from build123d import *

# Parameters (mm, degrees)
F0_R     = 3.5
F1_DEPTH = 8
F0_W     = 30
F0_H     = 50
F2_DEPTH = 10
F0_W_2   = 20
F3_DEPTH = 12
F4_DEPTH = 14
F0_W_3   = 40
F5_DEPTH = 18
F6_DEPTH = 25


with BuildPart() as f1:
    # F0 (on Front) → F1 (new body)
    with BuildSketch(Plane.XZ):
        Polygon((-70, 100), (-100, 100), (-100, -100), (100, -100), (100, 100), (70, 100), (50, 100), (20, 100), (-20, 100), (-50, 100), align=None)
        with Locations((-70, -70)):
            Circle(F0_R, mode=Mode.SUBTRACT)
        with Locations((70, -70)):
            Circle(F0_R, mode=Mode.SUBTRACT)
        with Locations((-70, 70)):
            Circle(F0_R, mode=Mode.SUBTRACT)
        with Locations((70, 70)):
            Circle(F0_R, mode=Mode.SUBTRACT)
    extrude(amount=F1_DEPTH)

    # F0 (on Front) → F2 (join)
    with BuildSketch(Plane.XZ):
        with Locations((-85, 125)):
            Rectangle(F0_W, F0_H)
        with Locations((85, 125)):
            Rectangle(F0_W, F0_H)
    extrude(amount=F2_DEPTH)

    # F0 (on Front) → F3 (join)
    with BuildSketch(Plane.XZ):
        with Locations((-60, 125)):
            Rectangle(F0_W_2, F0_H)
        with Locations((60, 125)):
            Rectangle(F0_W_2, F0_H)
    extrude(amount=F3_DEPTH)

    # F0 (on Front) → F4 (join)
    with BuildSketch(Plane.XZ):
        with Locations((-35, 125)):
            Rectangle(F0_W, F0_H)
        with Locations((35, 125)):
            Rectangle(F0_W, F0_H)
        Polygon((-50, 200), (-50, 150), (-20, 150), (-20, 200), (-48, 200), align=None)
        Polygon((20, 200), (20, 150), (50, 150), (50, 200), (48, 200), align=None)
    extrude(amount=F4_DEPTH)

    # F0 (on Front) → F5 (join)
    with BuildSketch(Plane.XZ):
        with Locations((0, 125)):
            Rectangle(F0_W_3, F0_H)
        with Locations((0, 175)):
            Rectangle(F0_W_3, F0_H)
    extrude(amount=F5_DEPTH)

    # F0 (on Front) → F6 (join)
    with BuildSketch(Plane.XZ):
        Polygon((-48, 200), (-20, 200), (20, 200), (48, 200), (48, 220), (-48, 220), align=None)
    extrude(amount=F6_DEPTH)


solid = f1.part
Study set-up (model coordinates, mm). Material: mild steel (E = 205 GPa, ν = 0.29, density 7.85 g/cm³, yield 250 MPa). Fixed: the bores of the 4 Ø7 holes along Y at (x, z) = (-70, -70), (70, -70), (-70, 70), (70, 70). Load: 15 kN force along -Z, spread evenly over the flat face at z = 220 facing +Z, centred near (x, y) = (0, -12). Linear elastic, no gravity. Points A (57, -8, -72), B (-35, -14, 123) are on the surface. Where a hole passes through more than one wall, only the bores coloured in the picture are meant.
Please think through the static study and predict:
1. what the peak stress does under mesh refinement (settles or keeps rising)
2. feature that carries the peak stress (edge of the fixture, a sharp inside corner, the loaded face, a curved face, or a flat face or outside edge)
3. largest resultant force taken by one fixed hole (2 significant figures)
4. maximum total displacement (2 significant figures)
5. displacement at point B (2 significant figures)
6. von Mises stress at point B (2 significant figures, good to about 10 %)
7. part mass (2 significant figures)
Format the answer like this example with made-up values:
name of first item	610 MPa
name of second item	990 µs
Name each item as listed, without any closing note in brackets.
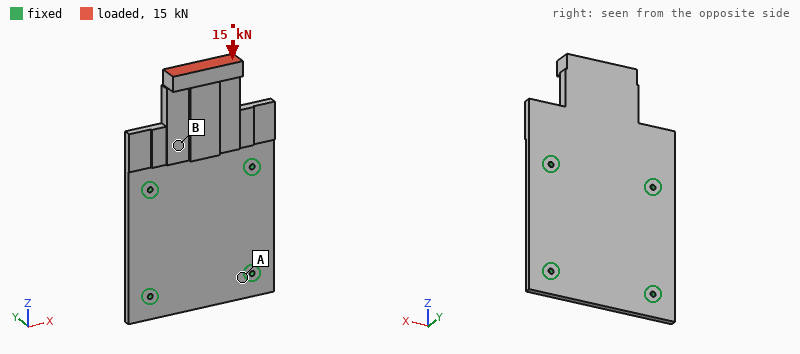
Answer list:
what the peak stress does under mesh refinement	keeps rising
feature that carries the peak stress	edge of the fixture
largest resultant force taken by one fixed hole	5.8 kN
maximum total displacement	0.50 mm
displacement at point B	0.13 mm
von Mises stress at point B	25 MPa
part mass	4.5 kg
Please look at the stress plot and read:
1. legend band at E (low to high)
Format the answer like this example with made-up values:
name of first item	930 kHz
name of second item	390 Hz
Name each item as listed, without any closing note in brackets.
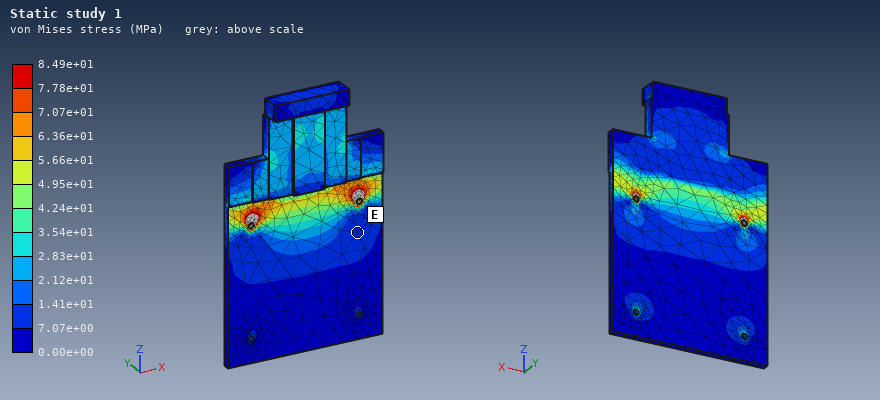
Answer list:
legend band at E	7.07e+00 to 1.41e+01 MPa
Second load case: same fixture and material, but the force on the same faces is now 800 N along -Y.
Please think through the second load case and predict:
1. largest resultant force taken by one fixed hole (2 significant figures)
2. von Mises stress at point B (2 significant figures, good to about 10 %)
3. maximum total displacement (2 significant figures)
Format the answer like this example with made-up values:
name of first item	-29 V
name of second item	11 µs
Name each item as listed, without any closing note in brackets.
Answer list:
largest resultant force taken by one fixed hole	610 N
von Mises stress at point B	16 MPa
maximum total displacement	0.43 mm
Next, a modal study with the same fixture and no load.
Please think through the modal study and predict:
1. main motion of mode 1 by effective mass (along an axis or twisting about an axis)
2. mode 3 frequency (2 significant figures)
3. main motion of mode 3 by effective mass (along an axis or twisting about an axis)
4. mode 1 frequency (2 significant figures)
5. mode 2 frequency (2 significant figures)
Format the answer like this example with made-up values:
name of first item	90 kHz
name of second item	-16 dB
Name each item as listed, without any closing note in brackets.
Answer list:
main motion of mode 1 by effective mass	along Y
mode 3 frequency	1400 Hz
main motion of mode 3 by effective mass	along Y
mode 1 frequency	260 Hz
mode 2 frequency	1300 Hz
